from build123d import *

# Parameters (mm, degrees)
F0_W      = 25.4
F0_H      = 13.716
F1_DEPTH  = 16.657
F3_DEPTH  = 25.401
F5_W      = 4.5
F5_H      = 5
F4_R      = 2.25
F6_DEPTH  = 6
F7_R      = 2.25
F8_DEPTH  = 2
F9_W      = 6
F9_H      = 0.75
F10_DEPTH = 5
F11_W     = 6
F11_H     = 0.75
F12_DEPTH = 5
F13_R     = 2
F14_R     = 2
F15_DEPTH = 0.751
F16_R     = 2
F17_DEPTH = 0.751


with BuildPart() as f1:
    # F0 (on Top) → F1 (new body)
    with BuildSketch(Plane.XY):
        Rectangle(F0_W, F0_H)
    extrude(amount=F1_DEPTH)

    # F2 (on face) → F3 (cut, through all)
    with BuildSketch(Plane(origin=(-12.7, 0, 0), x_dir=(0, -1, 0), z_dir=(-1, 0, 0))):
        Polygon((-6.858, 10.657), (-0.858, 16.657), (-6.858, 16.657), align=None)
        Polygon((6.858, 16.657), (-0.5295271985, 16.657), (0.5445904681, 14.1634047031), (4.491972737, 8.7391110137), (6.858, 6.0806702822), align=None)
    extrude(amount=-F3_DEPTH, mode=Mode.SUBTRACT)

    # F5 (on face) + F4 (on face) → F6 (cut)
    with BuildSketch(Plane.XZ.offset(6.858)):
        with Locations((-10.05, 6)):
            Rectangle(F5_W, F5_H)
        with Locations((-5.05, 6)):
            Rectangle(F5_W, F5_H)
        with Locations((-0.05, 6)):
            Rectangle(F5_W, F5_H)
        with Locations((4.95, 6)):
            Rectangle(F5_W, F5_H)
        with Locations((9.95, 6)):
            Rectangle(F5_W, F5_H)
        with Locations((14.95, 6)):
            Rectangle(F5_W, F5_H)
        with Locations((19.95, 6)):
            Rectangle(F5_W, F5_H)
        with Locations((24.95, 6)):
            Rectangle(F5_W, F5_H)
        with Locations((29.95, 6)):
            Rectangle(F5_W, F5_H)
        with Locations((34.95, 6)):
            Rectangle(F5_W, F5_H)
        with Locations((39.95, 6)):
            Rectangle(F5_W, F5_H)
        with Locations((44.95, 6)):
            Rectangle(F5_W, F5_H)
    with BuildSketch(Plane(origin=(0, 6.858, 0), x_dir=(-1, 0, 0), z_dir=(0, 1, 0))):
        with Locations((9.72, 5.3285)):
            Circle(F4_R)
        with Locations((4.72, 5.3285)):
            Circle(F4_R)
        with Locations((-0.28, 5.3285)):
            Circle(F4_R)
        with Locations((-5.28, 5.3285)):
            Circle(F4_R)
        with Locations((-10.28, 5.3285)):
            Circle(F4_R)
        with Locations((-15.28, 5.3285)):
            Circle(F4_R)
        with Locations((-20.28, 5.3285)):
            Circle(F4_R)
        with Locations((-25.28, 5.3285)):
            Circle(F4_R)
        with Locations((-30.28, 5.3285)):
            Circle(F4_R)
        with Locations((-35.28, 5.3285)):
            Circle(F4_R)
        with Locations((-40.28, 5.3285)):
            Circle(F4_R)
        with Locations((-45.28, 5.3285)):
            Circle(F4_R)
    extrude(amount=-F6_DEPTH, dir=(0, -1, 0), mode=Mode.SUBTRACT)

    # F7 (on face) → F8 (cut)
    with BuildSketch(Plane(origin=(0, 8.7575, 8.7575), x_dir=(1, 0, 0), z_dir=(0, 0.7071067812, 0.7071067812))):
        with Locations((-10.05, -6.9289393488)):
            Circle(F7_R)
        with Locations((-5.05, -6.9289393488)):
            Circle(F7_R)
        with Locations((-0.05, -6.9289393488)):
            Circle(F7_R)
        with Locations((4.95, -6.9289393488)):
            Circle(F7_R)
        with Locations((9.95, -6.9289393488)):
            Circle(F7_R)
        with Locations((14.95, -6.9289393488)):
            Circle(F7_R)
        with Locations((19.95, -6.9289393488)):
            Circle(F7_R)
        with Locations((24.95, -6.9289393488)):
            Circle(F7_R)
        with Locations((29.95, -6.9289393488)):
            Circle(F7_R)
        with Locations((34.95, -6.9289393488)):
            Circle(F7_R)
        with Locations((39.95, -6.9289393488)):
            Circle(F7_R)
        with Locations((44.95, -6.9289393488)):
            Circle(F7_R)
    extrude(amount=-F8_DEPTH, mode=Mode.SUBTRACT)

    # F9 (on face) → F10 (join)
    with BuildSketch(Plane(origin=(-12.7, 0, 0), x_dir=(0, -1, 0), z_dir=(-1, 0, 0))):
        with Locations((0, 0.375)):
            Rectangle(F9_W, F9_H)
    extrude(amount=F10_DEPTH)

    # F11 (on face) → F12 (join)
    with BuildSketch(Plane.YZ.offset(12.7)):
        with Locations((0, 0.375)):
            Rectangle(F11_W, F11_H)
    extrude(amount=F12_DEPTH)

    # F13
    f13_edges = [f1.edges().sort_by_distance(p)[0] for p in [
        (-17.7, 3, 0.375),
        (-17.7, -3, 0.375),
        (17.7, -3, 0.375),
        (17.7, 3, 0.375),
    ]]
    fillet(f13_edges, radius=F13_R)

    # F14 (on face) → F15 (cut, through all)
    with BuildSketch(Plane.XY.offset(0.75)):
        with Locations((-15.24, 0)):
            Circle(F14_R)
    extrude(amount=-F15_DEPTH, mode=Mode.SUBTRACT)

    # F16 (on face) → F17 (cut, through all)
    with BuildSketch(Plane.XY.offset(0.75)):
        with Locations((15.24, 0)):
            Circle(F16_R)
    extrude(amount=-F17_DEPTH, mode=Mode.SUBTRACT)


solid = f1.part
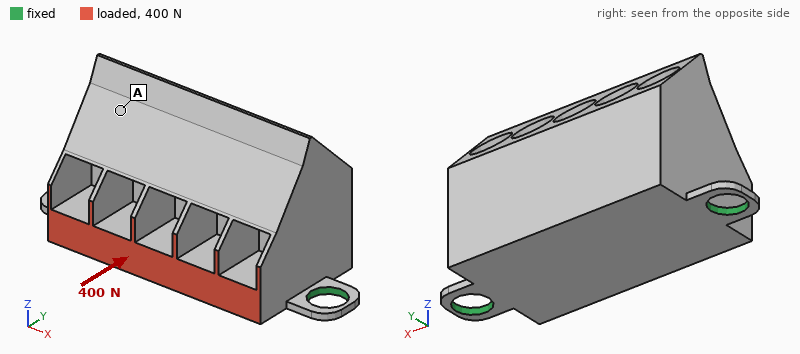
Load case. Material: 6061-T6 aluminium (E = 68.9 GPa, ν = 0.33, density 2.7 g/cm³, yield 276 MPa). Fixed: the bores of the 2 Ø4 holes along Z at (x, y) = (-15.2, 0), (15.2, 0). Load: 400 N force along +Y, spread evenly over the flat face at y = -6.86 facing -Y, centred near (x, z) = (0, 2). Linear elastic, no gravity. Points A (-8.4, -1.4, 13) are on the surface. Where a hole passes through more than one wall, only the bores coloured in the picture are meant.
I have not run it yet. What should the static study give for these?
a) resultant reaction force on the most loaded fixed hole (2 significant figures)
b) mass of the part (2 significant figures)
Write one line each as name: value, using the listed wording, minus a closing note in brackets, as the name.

resultant reaction force on the most loaded fixed hole: 200 N
mass of the part: 9.4 g
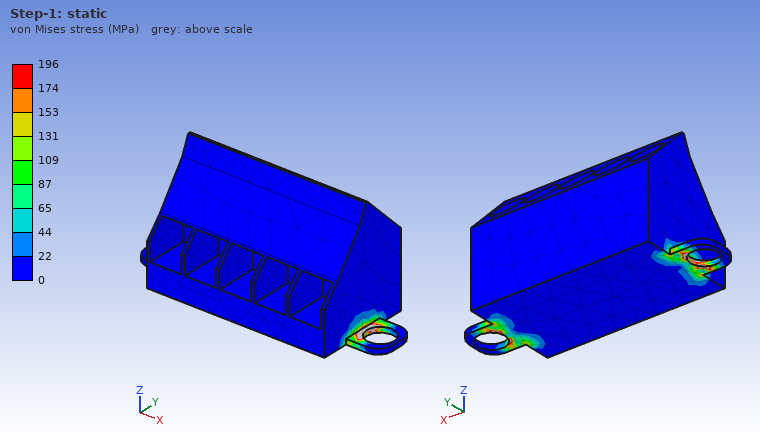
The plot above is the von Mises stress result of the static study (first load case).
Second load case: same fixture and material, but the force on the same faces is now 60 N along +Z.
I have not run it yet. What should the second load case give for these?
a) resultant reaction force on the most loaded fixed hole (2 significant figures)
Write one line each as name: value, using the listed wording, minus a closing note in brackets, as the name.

resultant reaction force on the most loaded fixed hole: 38 N
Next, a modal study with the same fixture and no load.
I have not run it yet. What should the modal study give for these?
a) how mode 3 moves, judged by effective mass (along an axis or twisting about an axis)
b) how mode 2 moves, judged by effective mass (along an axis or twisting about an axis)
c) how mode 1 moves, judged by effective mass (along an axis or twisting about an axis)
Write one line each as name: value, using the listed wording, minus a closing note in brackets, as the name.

how mode 3 moves, judged by effective mass: along X
how mode 2 moves, judged by effective mass: along Z
how mode 1 moves, judged by effective mass: along Y
